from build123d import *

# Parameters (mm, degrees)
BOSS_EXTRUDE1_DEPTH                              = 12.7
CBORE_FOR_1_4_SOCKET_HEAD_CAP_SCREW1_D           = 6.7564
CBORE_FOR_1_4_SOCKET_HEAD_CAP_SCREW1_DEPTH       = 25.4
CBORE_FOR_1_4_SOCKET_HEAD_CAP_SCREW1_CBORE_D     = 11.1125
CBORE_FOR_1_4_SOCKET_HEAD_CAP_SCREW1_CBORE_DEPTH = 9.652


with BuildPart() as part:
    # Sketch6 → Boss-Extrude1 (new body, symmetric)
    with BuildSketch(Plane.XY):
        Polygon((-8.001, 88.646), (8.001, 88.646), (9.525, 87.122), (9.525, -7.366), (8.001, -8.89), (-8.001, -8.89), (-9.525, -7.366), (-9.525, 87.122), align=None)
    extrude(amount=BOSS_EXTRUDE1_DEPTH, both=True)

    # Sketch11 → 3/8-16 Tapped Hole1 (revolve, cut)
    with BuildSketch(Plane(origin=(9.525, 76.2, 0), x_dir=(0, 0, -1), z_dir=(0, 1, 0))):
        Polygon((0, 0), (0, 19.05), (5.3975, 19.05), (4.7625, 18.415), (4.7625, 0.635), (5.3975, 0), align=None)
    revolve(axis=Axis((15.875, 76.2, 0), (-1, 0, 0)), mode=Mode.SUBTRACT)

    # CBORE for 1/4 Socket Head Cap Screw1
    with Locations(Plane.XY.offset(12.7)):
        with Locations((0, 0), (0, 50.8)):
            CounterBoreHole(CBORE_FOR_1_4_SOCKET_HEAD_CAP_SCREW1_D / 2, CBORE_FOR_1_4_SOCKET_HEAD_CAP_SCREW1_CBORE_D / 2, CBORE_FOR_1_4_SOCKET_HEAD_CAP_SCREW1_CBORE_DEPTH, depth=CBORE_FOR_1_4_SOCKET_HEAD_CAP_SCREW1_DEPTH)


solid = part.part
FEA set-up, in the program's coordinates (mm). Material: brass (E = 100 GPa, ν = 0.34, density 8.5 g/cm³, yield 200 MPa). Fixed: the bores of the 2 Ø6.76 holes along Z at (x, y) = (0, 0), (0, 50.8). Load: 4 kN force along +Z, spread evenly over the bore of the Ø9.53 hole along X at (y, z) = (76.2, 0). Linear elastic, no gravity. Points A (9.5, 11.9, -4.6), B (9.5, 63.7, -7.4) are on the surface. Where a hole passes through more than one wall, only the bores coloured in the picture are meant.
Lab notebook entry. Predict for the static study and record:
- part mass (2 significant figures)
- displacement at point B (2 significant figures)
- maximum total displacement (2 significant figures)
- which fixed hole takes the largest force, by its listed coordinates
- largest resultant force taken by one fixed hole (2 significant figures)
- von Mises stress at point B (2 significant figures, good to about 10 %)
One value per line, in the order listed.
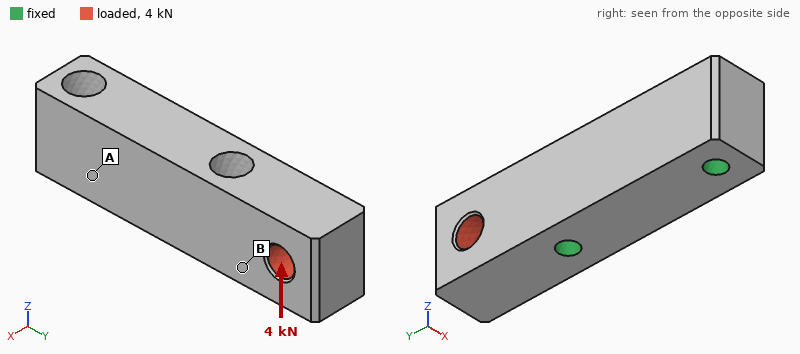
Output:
360 g
9.7 µm
40 µm
(0, 50.8)
4.9 kN
21 MPa
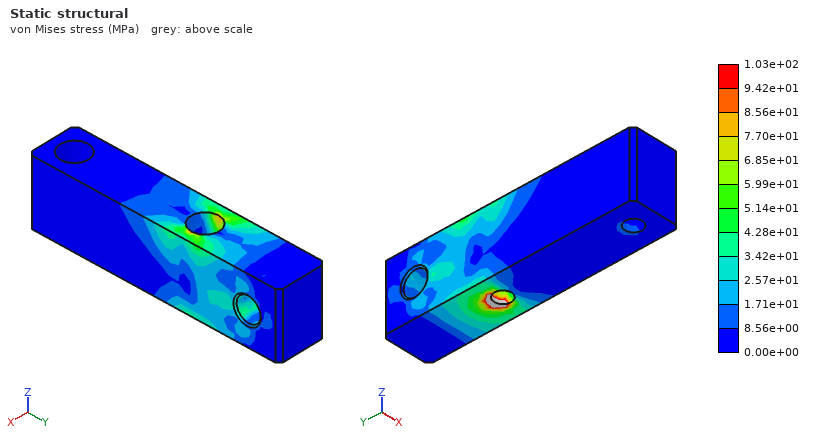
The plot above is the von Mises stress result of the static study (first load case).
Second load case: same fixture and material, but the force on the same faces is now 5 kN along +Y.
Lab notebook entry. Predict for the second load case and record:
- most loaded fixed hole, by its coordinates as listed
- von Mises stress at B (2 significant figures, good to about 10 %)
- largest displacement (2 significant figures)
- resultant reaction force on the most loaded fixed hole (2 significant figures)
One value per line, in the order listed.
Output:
(0, 50.8)
9.8 MPa
7.1 µm
4.4 kN
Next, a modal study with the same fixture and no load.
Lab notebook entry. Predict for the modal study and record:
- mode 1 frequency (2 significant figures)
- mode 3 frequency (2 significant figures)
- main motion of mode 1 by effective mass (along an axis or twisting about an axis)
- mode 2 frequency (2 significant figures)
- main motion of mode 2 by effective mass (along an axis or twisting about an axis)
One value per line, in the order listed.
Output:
5100 Hz
10000 Hz
along X
6000 Hz
along Z
